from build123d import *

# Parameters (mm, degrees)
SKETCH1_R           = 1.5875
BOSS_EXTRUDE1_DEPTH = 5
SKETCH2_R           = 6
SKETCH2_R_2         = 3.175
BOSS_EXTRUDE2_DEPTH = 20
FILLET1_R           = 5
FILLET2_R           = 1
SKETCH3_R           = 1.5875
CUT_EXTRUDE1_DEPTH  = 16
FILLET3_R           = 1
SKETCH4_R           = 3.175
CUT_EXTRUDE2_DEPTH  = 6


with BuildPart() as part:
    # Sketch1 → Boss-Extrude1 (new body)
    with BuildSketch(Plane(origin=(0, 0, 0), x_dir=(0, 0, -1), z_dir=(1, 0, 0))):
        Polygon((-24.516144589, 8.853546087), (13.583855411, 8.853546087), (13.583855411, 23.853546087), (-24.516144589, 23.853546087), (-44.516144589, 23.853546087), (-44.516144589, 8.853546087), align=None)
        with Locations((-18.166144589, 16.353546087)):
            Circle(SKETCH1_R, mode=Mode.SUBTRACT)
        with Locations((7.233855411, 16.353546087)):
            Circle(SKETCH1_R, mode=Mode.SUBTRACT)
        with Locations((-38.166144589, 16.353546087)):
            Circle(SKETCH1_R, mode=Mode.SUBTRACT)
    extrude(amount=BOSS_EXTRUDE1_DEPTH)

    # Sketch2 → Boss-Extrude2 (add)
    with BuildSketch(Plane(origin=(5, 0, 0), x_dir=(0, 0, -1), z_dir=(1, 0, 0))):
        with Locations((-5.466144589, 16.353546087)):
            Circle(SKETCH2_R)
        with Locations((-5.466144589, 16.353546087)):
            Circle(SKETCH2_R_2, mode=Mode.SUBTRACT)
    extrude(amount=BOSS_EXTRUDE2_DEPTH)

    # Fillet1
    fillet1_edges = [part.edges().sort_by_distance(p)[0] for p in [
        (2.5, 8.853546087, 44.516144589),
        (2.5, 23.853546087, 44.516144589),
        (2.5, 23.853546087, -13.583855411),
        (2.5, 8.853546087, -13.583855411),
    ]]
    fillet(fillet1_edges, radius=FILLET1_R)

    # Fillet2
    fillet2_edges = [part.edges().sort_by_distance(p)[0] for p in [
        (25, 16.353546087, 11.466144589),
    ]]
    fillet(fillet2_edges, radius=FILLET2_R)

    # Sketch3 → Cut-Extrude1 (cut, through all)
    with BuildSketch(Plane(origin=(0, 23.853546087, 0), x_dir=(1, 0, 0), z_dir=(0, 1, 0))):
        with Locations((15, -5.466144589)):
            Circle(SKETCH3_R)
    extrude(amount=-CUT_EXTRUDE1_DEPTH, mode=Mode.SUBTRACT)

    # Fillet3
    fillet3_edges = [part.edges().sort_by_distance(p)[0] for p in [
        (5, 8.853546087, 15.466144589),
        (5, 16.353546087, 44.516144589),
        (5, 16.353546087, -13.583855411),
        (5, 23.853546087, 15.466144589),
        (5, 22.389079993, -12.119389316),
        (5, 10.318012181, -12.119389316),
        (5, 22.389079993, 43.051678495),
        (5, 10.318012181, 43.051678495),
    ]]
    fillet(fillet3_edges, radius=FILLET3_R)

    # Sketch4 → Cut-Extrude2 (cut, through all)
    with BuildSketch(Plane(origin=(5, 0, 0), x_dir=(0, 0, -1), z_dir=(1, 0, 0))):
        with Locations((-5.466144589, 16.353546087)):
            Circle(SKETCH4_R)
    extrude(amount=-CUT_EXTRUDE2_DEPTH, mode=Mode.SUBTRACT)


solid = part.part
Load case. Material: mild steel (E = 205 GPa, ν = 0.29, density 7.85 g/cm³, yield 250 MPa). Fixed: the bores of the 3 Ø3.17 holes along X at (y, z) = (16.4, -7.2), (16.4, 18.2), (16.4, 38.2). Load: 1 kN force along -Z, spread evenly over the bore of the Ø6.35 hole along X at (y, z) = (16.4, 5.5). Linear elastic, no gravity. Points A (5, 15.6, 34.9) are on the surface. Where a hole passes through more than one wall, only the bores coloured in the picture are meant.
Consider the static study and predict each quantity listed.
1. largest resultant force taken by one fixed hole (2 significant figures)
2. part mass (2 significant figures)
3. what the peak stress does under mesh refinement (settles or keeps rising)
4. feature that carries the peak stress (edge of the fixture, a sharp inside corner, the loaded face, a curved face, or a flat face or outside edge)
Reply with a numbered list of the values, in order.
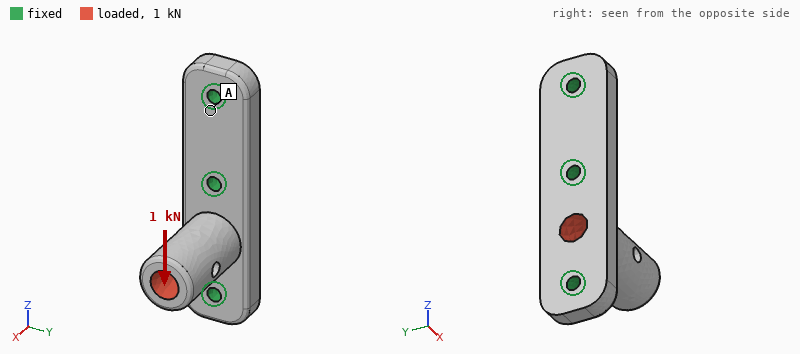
1. 710 N
2. 43 g
3. keeps rising
4. edge of the fixture
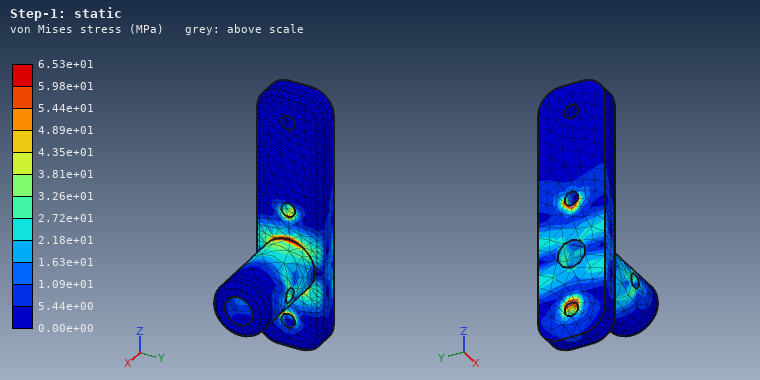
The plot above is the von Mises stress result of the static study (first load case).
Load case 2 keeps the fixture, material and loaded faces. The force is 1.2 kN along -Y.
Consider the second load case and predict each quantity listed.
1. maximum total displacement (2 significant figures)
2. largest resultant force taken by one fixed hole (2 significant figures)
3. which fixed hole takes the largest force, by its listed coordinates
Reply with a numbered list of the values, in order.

1. 41 µm
2. 730 N
3. (16.4, 18.2)
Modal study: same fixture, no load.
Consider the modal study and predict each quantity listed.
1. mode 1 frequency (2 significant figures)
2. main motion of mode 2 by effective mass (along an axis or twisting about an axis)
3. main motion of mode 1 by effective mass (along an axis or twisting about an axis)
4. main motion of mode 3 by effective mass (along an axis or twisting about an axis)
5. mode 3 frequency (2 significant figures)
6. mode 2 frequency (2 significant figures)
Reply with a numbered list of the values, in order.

1. 8200 Hz
2. along Z
3. along Y
4. along X
5. 22 kHz
6. 13 kHz
